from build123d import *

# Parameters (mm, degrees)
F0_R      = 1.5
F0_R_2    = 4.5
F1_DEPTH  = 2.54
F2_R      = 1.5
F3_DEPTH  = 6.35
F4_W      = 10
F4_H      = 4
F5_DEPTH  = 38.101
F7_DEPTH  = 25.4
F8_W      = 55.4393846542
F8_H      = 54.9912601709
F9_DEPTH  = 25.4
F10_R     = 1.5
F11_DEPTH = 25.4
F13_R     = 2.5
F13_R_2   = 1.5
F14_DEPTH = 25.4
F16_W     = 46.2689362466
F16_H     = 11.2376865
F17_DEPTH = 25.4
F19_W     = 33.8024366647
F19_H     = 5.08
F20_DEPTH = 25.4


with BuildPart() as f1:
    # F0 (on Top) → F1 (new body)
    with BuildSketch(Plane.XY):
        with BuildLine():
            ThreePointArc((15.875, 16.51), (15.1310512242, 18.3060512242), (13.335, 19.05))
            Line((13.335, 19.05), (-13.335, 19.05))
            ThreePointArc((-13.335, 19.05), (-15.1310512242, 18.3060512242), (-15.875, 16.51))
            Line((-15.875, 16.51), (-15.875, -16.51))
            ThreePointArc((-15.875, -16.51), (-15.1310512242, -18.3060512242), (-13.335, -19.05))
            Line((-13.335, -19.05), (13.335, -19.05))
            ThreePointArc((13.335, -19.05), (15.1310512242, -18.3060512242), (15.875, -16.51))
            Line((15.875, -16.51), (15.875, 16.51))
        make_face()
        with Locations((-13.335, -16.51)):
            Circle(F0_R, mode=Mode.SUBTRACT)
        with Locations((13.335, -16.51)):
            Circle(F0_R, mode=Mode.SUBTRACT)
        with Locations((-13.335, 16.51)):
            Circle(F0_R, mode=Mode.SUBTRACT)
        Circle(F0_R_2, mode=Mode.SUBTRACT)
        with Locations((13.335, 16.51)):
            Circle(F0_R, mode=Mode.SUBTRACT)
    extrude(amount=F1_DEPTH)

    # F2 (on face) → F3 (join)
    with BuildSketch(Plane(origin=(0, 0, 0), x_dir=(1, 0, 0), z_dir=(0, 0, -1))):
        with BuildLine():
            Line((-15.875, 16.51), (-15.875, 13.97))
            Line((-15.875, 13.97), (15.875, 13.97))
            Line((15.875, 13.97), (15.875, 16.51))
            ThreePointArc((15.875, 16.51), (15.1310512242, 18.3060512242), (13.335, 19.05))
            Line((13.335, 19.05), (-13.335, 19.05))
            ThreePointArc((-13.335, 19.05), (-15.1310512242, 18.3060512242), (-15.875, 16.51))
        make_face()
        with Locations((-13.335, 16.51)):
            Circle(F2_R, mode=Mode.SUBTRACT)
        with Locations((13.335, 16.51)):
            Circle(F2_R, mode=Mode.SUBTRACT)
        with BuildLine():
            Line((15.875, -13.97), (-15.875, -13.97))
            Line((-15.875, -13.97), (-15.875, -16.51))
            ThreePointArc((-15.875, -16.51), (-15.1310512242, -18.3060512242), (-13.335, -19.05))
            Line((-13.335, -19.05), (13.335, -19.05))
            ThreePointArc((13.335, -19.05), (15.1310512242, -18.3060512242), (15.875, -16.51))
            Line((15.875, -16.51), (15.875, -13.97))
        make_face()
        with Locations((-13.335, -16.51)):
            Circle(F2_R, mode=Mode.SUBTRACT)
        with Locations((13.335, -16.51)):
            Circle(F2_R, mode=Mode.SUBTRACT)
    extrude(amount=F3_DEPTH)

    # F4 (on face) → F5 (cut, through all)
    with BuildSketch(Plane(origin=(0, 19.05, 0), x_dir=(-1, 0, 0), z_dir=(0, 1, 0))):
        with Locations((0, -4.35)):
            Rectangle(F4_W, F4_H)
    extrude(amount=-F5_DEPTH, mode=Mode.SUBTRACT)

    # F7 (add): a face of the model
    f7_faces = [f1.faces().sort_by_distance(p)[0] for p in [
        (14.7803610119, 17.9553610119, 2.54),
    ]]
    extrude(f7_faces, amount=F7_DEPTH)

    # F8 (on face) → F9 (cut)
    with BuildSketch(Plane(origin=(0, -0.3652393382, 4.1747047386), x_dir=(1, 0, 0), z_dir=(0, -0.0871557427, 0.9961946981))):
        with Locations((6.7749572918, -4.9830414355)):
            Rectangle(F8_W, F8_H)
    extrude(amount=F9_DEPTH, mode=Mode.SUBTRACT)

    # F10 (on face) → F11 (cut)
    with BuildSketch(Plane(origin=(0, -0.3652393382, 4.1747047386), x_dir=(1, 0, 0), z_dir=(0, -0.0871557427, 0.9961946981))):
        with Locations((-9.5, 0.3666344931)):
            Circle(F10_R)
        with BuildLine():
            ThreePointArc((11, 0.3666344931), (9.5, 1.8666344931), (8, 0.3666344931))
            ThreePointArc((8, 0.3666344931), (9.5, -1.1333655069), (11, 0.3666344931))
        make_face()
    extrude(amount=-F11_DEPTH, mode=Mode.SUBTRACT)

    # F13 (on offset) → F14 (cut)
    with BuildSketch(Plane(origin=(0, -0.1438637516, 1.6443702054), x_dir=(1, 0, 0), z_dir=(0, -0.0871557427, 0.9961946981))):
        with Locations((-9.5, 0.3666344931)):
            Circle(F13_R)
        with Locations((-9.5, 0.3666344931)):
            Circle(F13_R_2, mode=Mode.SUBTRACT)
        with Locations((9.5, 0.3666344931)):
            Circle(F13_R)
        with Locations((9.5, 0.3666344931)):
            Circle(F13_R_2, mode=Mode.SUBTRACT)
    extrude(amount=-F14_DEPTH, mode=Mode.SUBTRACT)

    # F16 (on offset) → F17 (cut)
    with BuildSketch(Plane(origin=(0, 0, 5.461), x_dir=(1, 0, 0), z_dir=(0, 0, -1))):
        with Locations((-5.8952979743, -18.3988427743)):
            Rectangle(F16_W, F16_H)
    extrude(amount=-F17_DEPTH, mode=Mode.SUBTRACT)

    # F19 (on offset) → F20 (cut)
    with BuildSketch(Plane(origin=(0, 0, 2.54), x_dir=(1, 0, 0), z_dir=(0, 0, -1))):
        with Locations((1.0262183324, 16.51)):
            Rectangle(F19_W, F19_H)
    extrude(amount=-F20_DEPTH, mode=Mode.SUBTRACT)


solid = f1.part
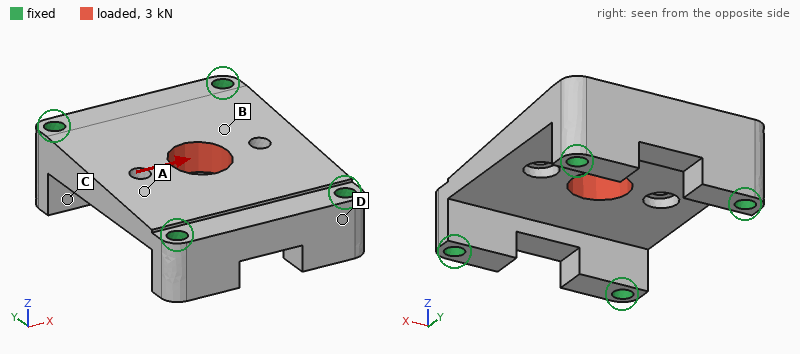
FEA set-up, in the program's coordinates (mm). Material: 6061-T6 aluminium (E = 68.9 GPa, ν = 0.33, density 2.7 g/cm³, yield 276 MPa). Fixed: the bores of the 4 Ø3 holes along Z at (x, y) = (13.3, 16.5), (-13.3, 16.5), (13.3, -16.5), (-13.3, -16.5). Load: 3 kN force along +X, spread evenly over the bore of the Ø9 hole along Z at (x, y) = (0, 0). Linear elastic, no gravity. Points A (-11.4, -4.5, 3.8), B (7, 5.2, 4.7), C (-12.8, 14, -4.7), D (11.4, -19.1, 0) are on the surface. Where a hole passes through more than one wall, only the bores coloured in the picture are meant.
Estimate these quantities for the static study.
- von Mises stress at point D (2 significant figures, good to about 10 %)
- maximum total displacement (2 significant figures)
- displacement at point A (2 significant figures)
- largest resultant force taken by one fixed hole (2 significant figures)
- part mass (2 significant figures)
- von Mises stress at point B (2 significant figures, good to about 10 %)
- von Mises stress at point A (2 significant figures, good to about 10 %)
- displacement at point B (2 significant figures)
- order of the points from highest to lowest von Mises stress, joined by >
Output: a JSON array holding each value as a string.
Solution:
["7.4 MPa", "9.9 µm", "6.9 µm", "1.0 kN", "16 g", "19 MPa", "16 MPa", "5.7 µm", "B > A > D > C"]
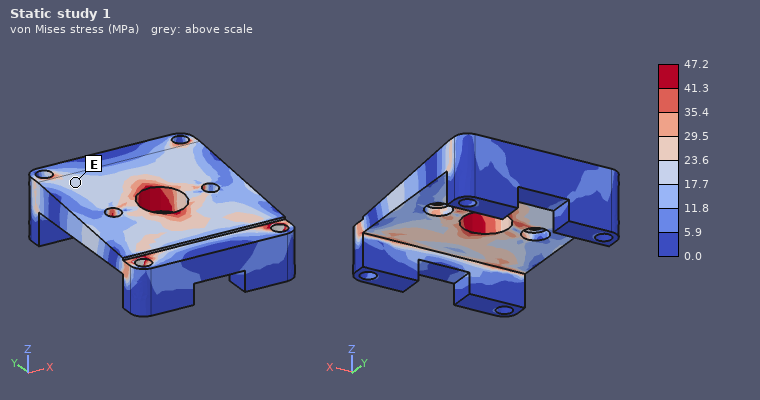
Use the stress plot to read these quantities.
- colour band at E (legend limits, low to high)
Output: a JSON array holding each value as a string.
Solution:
["17.7 to 23.6 MPa"]
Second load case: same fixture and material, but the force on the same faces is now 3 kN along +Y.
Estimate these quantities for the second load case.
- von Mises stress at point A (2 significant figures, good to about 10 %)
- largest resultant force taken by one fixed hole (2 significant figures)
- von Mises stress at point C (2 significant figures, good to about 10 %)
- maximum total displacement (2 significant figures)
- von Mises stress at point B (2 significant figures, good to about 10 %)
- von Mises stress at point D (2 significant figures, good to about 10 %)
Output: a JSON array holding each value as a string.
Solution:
["10 MPa", "1.0 kN", "8.9 MPa", "9.9 µm", "14 MPa", "19 MPa"]
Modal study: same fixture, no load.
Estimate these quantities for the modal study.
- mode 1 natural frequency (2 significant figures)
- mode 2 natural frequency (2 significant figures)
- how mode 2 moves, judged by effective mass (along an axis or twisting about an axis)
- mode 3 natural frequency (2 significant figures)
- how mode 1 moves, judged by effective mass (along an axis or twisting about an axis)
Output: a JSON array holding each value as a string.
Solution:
["18 kHz", "23 kHz", "twisting about Y", "33 kHz", "along Z"]
